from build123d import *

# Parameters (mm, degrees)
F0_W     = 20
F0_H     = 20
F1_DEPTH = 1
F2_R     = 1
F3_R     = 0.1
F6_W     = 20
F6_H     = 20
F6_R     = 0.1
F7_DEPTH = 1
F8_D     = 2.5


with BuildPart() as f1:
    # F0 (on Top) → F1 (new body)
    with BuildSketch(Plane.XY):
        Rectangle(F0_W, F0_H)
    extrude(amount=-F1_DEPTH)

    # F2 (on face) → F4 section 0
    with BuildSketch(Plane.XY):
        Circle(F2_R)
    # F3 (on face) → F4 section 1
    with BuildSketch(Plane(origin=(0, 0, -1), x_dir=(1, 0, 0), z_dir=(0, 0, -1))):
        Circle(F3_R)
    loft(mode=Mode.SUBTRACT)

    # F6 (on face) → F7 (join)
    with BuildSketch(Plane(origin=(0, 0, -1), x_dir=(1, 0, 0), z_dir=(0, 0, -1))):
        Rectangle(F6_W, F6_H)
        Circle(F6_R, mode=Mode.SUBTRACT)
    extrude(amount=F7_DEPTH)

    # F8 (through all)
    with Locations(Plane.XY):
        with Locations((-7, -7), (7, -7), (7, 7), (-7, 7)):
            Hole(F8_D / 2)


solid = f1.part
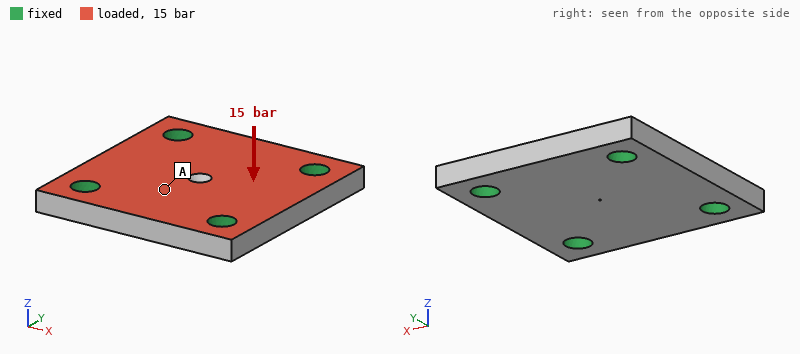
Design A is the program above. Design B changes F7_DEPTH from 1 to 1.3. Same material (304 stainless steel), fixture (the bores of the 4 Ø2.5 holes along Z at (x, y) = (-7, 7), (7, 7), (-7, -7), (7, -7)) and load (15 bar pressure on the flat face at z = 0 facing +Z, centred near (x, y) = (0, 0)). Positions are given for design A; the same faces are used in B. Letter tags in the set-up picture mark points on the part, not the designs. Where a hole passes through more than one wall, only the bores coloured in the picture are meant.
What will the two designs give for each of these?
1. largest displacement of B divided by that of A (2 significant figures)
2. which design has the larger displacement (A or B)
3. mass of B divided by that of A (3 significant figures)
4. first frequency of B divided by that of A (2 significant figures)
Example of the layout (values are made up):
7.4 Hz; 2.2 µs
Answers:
0.71; A; 1.15; 1.1
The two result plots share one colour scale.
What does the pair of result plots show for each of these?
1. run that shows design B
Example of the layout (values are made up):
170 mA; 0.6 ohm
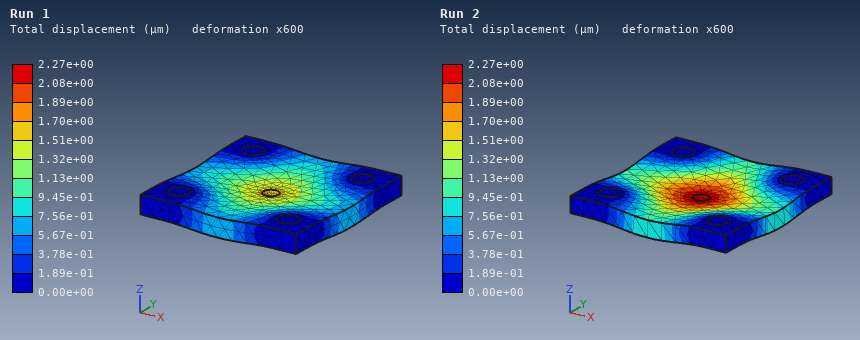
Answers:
Run 1
